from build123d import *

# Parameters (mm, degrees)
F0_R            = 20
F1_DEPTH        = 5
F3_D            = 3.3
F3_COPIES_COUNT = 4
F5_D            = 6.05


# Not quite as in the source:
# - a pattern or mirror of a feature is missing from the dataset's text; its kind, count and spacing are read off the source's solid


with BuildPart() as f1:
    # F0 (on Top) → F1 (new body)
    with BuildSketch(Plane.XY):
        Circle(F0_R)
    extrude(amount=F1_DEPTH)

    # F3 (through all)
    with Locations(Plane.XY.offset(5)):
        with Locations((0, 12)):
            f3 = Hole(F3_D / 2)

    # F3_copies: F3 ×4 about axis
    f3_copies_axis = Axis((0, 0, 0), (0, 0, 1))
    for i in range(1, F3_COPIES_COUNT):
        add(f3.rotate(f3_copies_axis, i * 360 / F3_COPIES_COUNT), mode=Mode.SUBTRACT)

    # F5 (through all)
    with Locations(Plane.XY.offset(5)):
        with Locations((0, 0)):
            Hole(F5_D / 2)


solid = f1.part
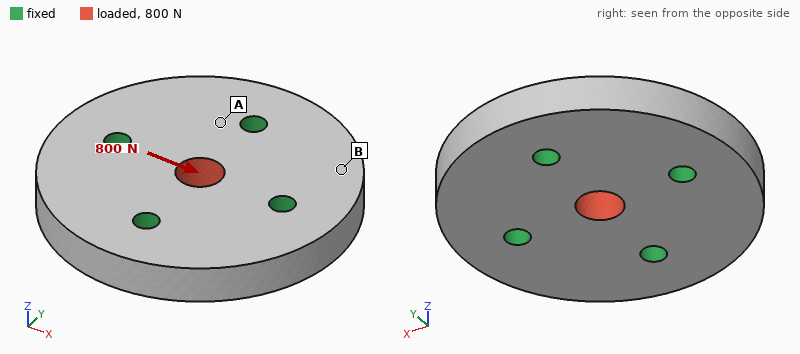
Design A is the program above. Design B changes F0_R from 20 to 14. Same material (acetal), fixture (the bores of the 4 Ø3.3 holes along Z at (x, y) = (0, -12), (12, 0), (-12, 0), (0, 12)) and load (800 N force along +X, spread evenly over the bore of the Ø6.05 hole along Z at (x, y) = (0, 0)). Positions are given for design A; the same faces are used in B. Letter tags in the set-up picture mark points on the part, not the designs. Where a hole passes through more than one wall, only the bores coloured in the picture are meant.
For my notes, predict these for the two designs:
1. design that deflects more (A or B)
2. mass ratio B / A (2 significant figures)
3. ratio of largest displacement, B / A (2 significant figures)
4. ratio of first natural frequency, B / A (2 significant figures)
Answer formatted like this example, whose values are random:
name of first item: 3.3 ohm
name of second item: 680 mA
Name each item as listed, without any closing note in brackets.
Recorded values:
design that deflects more: B
mass ratio B / A: 0.46
ratio of largest displacement, B / A: 1.1
ratio of first natural frequency, B / A: 1.9
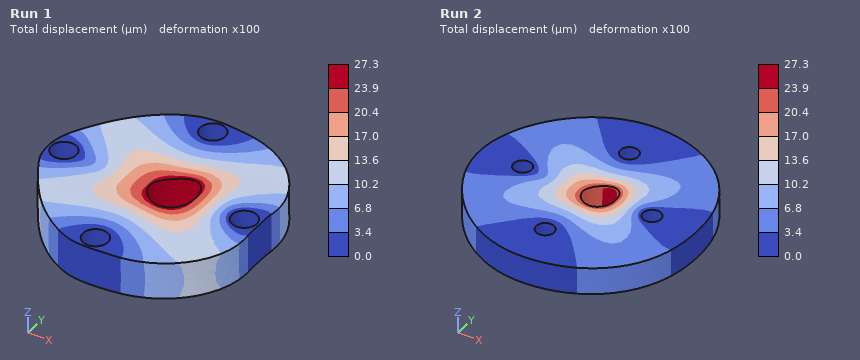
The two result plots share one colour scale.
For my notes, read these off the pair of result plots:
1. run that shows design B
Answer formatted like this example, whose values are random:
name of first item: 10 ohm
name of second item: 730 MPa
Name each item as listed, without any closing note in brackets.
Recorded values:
run that shows design B: Run 1
